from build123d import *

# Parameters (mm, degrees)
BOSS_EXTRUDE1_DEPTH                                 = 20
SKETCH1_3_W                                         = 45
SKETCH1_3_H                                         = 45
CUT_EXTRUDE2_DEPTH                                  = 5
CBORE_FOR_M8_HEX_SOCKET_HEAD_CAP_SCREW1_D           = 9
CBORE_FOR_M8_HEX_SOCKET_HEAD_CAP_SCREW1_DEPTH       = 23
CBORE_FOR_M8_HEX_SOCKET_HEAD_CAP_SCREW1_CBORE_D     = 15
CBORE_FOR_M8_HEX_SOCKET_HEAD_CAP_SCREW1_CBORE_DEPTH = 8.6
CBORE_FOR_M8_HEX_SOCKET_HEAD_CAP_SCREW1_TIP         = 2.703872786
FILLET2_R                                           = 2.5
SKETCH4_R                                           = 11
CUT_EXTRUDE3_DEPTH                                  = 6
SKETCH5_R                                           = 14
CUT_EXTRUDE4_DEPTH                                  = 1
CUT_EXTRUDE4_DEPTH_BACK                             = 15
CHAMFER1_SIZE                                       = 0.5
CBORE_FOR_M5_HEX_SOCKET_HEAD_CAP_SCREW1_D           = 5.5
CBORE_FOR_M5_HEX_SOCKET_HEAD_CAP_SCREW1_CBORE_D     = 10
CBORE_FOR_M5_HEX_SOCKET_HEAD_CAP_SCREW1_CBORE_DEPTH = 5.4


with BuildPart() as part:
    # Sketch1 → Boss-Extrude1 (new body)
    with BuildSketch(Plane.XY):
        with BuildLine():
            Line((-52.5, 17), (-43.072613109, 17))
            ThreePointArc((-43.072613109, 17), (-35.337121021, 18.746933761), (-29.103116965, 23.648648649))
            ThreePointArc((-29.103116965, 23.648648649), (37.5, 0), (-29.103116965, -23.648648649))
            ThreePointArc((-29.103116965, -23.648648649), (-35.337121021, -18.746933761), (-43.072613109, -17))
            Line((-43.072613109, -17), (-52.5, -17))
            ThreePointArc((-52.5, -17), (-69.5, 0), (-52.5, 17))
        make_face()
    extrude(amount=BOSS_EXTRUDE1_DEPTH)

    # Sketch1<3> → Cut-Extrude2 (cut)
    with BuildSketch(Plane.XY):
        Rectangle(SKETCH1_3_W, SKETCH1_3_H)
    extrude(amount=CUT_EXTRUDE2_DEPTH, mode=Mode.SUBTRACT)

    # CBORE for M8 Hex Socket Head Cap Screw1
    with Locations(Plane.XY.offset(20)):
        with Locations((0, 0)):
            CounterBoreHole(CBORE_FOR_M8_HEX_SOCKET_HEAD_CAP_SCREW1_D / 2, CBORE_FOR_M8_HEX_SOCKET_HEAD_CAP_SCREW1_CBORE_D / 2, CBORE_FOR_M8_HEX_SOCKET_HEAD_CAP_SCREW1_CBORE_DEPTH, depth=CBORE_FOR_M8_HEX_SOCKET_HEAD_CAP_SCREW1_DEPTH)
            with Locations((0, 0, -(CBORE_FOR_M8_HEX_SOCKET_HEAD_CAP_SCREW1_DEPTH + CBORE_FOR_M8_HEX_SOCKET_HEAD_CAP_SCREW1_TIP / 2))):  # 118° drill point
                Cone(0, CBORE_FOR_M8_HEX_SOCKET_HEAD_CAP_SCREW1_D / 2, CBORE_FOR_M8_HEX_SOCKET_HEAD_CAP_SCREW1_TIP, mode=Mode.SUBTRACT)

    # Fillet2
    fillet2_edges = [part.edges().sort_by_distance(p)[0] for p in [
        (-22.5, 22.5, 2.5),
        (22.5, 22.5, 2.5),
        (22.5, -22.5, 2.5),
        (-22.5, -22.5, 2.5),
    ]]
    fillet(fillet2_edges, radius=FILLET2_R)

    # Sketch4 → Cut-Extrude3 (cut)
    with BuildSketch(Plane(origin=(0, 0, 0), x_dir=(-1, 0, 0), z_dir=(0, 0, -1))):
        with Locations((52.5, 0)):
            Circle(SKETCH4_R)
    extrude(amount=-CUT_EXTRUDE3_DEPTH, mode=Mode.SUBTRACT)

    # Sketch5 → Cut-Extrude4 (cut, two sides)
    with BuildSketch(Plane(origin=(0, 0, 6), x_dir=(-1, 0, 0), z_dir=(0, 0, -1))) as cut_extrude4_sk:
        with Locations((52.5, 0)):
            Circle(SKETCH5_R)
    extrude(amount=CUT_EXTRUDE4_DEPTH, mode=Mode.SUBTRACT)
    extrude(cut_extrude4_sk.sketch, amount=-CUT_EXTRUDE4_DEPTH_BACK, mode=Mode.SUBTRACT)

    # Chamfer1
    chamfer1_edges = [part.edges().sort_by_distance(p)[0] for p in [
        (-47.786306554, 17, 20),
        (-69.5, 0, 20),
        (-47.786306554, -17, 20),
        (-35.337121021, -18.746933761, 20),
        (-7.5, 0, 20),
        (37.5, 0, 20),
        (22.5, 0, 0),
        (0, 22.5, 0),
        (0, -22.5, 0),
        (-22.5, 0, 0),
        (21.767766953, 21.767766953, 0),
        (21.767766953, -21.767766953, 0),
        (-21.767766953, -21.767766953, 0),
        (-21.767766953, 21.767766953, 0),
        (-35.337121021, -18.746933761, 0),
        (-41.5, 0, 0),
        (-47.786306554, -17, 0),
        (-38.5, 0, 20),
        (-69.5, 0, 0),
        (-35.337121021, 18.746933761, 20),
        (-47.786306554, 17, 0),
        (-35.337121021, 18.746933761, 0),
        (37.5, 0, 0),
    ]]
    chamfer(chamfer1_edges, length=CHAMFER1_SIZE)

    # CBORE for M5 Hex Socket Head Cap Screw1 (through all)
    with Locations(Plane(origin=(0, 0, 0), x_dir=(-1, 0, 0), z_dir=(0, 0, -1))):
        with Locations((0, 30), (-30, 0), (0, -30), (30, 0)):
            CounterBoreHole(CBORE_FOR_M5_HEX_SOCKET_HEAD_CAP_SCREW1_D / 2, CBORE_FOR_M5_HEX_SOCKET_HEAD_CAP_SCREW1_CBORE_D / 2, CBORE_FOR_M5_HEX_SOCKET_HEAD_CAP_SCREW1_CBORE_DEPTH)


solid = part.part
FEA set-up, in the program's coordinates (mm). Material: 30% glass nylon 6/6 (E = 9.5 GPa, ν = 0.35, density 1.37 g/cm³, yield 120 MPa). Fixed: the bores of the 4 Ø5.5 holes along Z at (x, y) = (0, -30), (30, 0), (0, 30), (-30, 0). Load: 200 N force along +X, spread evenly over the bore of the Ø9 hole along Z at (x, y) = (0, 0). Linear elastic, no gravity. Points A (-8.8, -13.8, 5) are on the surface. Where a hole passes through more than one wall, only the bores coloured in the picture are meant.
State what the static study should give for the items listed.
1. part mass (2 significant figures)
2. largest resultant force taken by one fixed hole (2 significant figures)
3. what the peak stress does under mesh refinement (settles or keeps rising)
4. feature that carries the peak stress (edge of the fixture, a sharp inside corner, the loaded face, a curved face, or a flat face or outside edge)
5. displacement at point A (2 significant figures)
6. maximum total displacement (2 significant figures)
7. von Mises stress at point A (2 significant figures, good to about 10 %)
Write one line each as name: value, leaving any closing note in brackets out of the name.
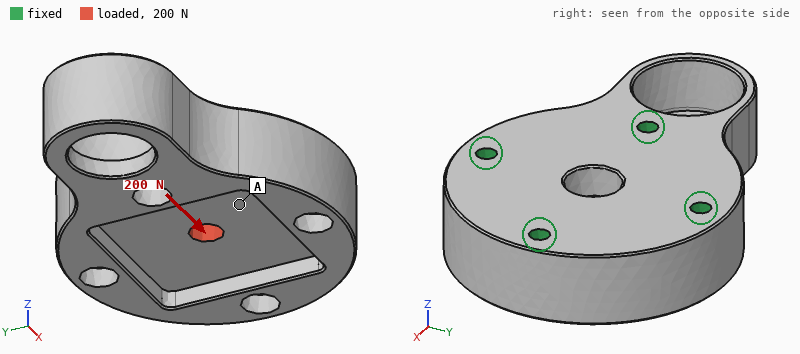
part mass: 110 g
largest resultant force taken by one fixed hole: 68 N
what the peak stress does under mesh refinement: keeps rising
feature that carries the peak stress: a sharp inside corner
displacement at point A: 0.47 µm
maximum total displacement: 1.6 µm
von Mises stress at point A: 0.19 MPa
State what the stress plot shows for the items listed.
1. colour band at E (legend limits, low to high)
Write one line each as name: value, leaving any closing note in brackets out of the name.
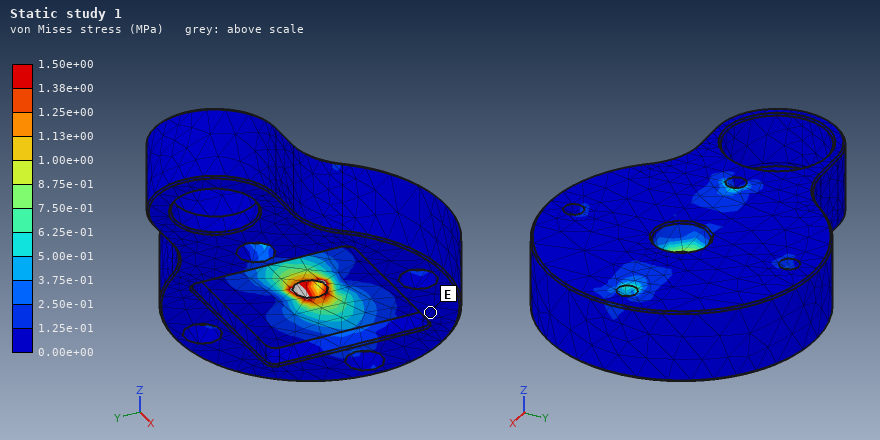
colour band at E: 0.00e+00 to 1.25e-01 MPa
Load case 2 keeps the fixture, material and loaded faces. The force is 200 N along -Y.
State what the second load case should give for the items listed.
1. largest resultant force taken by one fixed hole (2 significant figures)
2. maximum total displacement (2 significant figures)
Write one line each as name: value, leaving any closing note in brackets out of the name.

largest resultant force taken by one fixed hole: 67 N
maximum total displacement: 1.6 µm
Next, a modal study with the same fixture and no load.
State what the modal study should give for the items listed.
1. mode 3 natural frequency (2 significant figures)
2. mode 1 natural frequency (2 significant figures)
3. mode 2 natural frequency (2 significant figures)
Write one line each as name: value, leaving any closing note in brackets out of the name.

mode 3 natural frequency: 6800 Hz
mode 1 natural frequency: 4000 Hz
mode 2 natural frequency: 4200 Hz
